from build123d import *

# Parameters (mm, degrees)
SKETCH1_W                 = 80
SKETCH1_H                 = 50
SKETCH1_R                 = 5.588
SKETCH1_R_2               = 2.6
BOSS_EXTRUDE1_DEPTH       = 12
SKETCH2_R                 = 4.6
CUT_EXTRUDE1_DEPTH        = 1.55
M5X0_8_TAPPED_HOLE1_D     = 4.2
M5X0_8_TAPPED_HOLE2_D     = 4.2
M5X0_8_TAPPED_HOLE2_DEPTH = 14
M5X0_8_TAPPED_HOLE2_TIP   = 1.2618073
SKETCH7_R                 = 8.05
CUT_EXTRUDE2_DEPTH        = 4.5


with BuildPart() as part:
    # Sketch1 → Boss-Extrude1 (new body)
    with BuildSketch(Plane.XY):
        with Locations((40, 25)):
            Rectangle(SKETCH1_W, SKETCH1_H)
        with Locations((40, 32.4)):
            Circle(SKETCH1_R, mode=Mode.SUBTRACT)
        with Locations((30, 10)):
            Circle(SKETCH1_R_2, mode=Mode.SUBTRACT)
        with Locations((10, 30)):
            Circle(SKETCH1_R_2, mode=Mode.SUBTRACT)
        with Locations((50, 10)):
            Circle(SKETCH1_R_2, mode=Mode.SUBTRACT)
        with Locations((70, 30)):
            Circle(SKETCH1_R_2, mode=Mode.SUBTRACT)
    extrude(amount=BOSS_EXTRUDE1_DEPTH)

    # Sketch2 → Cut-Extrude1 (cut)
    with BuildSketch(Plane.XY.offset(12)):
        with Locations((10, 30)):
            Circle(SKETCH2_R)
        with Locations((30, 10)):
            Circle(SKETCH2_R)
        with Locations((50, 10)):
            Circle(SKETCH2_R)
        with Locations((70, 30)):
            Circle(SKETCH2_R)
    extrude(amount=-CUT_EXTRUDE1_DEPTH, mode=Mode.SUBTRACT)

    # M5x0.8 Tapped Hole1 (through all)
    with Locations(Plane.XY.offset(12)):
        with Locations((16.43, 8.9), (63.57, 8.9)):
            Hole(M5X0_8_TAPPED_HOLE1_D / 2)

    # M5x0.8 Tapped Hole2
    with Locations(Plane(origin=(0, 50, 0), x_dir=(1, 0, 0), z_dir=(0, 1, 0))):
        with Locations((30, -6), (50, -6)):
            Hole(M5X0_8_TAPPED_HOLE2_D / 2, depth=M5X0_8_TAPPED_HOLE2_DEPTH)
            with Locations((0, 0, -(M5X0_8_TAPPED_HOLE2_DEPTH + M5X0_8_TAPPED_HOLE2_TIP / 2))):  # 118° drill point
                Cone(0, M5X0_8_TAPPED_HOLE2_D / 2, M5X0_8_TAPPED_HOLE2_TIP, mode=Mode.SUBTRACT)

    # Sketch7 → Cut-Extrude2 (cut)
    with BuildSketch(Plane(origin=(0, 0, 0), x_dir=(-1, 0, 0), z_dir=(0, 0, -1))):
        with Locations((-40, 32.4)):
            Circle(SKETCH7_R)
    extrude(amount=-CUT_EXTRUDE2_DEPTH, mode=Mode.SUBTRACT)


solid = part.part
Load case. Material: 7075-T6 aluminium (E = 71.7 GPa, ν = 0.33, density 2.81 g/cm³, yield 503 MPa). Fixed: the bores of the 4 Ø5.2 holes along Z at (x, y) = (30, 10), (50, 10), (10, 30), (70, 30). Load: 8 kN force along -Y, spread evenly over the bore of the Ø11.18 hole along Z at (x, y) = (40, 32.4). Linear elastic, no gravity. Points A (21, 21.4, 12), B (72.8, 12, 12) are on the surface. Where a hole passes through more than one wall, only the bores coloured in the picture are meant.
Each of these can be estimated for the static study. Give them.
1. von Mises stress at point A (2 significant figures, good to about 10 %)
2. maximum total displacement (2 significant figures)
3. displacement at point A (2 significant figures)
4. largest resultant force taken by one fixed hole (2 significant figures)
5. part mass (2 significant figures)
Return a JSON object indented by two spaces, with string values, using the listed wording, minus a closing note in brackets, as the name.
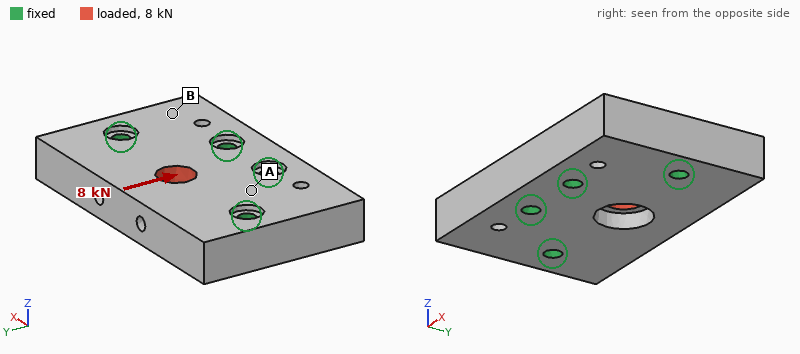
{
  "von Mises stress at point A": "9.1 MPa",
  "maximum total displacement": "15 µm",
  "displacement at point A": "2.8 µm",
  "largest resultant force taken by one fixed hole": "3.1 kN",
  "part mass": "120 g"
}
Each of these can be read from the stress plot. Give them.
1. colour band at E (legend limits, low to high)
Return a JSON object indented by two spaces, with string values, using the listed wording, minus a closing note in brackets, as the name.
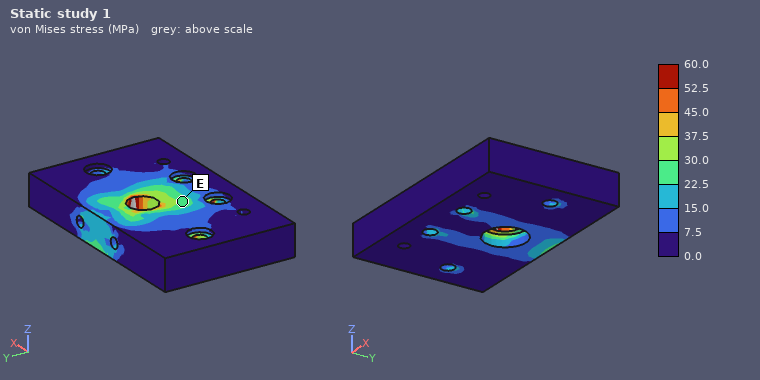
{
  "colour band at E": "22.5 to 30.0 MPa"
}
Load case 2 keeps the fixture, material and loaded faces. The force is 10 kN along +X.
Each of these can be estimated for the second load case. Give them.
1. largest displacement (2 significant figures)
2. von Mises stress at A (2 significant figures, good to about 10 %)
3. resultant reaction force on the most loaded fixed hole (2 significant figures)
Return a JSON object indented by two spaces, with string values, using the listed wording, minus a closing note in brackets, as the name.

{
  "largest displacement": "12 µm",
  "von Mises stress at A": "9.6 MPa",
  "resultant reaction force on the most loaded fixed hole": "3.8 kN"
}
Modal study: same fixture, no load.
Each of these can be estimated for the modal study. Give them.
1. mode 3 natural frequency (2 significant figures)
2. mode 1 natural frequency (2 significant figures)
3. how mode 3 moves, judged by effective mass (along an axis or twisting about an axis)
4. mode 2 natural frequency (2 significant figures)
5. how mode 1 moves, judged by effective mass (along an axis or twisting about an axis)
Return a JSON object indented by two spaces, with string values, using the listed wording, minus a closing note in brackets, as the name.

{
  "mode 3 natural frequency": "16 kHz",
  "mode 1 natural frequency": "11 kHz",
  "how mode 3 moves, judged by effective mass": "along Z",
  "mode 2 natural frequency": "15 kHz",
  "how mode 1 moves, judged by effective mass": "along Z"
}
